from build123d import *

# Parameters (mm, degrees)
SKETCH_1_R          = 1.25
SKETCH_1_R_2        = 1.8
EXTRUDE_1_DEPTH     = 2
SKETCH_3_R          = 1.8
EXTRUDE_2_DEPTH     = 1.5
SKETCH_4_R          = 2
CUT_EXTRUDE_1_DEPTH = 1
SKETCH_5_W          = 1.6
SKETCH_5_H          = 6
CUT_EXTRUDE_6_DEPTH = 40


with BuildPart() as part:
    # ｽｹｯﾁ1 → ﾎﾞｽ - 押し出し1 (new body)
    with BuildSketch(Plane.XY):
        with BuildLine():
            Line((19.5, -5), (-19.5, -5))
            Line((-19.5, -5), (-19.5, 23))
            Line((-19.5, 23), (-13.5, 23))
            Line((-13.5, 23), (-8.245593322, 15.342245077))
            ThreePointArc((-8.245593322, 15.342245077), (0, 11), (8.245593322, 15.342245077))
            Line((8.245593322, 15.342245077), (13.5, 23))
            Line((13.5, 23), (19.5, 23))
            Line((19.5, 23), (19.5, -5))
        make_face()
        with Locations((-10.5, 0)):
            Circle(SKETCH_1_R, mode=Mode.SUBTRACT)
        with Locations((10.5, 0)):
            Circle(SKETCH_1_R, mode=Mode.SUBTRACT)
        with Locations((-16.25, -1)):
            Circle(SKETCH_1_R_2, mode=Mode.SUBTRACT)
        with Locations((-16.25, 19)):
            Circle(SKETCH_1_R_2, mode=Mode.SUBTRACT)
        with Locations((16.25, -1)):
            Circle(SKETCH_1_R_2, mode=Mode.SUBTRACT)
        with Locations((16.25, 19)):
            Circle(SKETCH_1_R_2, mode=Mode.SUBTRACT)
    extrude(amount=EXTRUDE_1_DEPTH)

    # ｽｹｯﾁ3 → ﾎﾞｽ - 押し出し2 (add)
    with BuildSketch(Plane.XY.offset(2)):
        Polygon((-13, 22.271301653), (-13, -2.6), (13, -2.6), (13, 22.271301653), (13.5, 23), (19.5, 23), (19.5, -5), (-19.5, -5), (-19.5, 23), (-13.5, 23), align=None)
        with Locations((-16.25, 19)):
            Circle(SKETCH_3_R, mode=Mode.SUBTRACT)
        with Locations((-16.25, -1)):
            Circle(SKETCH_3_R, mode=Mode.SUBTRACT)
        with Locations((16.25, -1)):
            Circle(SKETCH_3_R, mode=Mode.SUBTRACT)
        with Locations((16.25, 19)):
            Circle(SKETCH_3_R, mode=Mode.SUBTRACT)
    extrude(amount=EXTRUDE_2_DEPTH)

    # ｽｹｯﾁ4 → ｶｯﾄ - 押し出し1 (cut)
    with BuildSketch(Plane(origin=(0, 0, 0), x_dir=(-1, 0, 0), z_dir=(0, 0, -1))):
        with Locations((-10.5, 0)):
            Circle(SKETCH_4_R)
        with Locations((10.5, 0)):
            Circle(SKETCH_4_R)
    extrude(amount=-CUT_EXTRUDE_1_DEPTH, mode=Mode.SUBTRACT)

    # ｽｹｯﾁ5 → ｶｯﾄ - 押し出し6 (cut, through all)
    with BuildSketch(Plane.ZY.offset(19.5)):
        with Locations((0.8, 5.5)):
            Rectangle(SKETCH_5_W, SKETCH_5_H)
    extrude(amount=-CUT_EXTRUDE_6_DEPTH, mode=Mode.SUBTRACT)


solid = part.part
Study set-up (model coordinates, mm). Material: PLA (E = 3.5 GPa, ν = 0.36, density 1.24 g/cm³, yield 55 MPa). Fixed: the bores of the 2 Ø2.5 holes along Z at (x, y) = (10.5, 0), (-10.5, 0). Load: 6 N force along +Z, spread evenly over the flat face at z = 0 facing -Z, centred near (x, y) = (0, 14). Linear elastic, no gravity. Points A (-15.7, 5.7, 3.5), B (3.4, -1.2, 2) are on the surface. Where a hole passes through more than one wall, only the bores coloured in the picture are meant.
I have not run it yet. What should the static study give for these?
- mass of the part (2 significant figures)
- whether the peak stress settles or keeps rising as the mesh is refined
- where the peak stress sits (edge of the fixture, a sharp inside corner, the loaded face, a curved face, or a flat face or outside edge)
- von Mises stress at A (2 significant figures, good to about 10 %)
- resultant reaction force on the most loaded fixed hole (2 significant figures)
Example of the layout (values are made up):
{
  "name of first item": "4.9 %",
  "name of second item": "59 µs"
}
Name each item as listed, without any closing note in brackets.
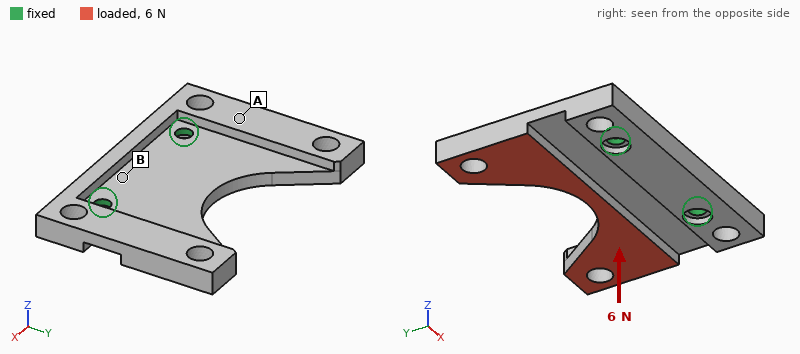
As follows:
{
  "mass of the part": "2.3 g",
  "whether the peak stress settles or keeps rising as the mesh is refined": "keeps rising",
  "where the peak stress sits": "edge of the fixture",
  "von Mises stress at A": "5.8 MPa",
  "resultant reaction force on the most loaded fixed hole": "3.3 N"
}
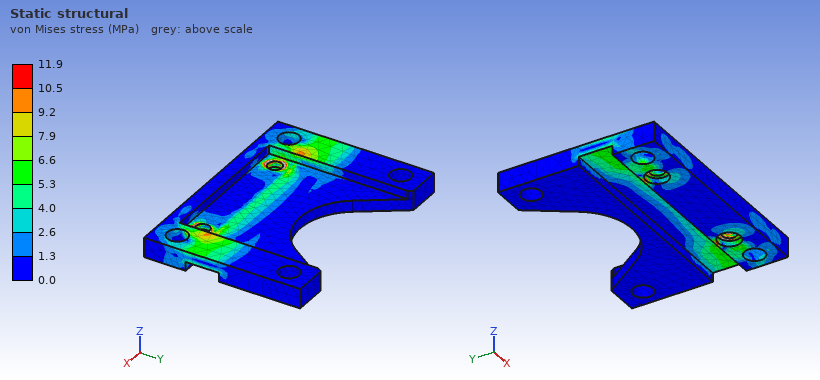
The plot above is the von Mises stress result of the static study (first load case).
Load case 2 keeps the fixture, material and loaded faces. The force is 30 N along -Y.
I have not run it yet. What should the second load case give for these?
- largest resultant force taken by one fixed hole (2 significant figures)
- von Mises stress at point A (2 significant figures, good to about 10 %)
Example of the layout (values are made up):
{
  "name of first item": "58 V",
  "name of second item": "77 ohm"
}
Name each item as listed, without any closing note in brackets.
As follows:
{
  "largest resultant force taken by one fixed hole": "15 N",
  "von Mises stress at point A": "6.7 MPa"
}
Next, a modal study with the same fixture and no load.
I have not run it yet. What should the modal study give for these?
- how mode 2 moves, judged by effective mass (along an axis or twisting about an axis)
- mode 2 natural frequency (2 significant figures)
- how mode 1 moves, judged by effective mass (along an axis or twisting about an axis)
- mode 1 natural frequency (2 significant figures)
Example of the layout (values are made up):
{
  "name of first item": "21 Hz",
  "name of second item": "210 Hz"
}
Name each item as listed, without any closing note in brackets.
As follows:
{
  "how mode 2 moves, judged by effective mass": "twisting about Y",
  "mode 2 natural frequency": "840 Hz",
  "how mode 1 moves, judged by effective mass": "along Z",
  "mode 1 natural frequency": "650 Hz"
}
